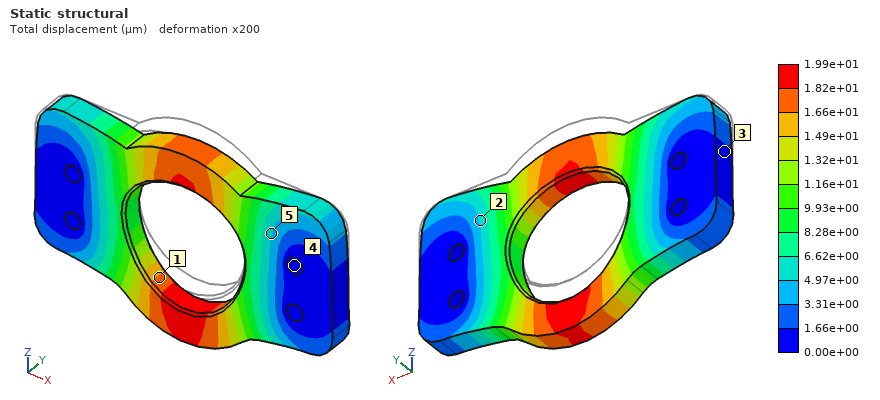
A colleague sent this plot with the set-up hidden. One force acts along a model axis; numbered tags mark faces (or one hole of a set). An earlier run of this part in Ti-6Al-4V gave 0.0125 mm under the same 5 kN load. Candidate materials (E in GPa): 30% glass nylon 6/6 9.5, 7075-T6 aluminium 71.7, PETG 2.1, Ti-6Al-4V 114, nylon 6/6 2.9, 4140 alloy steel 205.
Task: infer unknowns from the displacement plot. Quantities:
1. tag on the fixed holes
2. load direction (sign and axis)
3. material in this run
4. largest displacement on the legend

4
-Z
7075-T6 aluminium
1.99e+01 µm
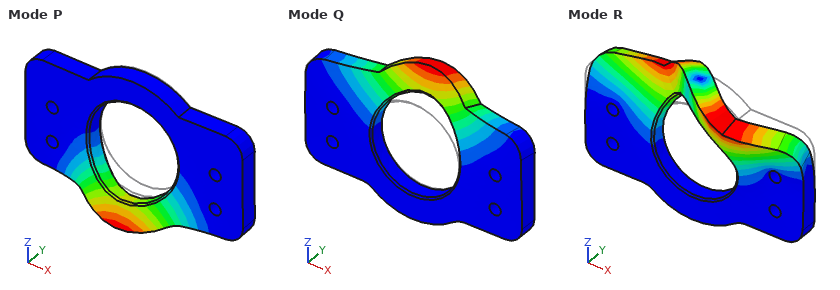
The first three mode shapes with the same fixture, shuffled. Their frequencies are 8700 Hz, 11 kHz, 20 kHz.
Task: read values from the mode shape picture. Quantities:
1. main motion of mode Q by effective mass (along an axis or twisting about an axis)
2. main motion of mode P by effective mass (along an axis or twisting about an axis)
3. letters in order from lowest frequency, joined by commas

along Y
along Y
Q, P, R
